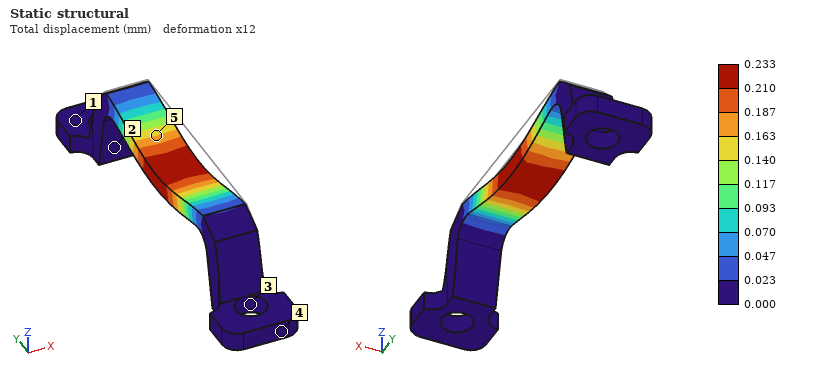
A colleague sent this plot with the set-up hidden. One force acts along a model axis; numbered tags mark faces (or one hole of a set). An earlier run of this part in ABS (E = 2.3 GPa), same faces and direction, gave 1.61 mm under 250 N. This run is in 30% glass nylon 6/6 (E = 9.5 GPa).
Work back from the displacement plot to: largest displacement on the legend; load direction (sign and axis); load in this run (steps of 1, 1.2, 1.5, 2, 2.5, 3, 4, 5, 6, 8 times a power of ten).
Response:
0.233 mm
-Z
150 N
